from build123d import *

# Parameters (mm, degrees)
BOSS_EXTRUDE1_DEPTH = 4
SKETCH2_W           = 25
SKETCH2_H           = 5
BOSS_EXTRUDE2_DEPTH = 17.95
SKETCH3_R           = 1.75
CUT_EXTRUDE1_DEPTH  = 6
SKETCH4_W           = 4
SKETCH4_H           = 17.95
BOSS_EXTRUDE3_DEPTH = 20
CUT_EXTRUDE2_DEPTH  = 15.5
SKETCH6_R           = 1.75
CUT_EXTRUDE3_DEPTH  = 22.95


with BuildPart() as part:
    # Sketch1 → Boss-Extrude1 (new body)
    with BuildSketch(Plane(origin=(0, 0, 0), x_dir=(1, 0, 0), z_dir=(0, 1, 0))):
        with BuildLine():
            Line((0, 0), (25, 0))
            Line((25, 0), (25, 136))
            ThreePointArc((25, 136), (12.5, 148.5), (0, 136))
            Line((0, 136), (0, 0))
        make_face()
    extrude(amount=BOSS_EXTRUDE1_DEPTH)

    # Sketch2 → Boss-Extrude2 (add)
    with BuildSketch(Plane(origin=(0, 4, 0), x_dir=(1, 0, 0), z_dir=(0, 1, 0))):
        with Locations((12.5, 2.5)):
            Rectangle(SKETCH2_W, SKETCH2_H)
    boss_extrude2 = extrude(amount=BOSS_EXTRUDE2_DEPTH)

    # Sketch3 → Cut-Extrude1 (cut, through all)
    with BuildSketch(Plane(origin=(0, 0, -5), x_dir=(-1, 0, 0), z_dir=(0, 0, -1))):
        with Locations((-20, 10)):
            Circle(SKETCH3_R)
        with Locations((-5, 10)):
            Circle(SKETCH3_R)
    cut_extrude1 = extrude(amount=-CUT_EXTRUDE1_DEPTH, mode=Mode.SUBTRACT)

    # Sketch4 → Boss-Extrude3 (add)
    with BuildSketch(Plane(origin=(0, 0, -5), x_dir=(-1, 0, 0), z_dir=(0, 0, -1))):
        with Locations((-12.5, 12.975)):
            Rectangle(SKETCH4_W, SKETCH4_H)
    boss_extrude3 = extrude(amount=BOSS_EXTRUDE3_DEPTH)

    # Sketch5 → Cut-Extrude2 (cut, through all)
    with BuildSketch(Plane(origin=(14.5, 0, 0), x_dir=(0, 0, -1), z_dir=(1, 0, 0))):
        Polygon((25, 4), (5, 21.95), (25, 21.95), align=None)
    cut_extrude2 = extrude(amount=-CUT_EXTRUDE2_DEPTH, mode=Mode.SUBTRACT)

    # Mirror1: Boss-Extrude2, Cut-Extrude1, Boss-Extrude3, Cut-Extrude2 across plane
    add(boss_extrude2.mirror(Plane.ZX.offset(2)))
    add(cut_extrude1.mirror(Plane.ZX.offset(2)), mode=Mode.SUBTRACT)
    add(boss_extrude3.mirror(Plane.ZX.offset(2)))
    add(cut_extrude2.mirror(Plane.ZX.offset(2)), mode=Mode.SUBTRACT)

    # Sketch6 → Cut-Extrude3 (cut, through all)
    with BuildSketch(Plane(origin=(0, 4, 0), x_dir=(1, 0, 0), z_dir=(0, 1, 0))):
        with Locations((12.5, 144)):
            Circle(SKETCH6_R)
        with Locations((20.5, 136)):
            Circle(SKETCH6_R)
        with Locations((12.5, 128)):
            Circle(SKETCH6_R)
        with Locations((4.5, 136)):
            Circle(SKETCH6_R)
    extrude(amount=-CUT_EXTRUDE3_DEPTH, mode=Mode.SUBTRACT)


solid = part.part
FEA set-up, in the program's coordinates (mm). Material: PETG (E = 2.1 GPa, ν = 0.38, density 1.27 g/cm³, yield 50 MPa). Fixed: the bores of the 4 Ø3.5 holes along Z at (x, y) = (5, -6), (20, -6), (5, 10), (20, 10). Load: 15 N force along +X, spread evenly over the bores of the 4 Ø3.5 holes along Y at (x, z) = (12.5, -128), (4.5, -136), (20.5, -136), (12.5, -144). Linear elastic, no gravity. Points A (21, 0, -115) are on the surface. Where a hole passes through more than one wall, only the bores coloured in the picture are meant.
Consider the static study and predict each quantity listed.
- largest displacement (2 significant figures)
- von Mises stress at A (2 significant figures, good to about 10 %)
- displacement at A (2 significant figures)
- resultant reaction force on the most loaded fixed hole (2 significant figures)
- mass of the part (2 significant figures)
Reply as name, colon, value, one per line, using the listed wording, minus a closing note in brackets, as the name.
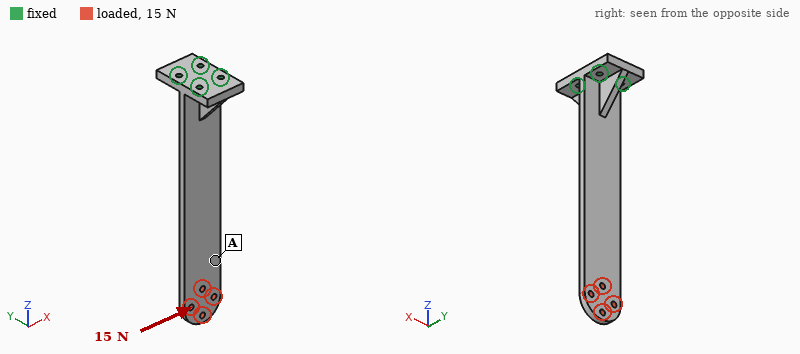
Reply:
largest displacement: 1.5 mm
von Mises stress at A: 0.58 MPa
displacement at A: 1.0 mm
resultant reaction force on the most loaded fixed hole: 59 N
mass of the part: 26 g
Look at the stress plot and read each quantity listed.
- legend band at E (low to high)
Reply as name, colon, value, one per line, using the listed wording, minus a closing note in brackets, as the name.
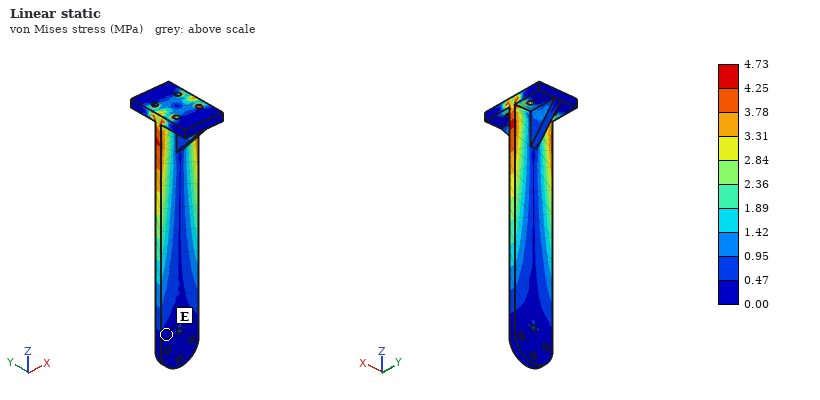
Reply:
legend band at E: 0.00 to 0.47 MPa
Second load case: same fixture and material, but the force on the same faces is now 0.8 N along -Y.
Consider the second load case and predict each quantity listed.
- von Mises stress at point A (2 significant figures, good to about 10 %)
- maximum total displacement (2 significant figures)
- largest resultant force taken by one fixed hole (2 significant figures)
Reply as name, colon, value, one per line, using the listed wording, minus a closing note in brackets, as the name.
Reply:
von Mises stress at point A: 0.26 MPa
maximum total displacement: 1.7 mm
largest resultant force taken by one fixed hole: 2.5 N
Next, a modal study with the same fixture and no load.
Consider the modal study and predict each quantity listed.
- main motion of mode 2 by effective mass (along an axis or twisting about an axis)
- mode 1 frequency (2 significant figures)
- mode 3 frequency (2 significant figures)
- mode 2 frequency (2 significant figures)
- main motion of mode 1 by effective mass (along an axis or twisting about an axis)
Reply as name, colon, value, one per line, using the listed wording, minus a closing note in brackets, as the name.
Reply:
main motion of mode 2 by effective mass: along X
mode 1 frequency: 54 Hz
mode 3 frequency: 330 Hz
mode 2 frequency: 230 Hz
main motion of mode 1 by effective mass: along Y
